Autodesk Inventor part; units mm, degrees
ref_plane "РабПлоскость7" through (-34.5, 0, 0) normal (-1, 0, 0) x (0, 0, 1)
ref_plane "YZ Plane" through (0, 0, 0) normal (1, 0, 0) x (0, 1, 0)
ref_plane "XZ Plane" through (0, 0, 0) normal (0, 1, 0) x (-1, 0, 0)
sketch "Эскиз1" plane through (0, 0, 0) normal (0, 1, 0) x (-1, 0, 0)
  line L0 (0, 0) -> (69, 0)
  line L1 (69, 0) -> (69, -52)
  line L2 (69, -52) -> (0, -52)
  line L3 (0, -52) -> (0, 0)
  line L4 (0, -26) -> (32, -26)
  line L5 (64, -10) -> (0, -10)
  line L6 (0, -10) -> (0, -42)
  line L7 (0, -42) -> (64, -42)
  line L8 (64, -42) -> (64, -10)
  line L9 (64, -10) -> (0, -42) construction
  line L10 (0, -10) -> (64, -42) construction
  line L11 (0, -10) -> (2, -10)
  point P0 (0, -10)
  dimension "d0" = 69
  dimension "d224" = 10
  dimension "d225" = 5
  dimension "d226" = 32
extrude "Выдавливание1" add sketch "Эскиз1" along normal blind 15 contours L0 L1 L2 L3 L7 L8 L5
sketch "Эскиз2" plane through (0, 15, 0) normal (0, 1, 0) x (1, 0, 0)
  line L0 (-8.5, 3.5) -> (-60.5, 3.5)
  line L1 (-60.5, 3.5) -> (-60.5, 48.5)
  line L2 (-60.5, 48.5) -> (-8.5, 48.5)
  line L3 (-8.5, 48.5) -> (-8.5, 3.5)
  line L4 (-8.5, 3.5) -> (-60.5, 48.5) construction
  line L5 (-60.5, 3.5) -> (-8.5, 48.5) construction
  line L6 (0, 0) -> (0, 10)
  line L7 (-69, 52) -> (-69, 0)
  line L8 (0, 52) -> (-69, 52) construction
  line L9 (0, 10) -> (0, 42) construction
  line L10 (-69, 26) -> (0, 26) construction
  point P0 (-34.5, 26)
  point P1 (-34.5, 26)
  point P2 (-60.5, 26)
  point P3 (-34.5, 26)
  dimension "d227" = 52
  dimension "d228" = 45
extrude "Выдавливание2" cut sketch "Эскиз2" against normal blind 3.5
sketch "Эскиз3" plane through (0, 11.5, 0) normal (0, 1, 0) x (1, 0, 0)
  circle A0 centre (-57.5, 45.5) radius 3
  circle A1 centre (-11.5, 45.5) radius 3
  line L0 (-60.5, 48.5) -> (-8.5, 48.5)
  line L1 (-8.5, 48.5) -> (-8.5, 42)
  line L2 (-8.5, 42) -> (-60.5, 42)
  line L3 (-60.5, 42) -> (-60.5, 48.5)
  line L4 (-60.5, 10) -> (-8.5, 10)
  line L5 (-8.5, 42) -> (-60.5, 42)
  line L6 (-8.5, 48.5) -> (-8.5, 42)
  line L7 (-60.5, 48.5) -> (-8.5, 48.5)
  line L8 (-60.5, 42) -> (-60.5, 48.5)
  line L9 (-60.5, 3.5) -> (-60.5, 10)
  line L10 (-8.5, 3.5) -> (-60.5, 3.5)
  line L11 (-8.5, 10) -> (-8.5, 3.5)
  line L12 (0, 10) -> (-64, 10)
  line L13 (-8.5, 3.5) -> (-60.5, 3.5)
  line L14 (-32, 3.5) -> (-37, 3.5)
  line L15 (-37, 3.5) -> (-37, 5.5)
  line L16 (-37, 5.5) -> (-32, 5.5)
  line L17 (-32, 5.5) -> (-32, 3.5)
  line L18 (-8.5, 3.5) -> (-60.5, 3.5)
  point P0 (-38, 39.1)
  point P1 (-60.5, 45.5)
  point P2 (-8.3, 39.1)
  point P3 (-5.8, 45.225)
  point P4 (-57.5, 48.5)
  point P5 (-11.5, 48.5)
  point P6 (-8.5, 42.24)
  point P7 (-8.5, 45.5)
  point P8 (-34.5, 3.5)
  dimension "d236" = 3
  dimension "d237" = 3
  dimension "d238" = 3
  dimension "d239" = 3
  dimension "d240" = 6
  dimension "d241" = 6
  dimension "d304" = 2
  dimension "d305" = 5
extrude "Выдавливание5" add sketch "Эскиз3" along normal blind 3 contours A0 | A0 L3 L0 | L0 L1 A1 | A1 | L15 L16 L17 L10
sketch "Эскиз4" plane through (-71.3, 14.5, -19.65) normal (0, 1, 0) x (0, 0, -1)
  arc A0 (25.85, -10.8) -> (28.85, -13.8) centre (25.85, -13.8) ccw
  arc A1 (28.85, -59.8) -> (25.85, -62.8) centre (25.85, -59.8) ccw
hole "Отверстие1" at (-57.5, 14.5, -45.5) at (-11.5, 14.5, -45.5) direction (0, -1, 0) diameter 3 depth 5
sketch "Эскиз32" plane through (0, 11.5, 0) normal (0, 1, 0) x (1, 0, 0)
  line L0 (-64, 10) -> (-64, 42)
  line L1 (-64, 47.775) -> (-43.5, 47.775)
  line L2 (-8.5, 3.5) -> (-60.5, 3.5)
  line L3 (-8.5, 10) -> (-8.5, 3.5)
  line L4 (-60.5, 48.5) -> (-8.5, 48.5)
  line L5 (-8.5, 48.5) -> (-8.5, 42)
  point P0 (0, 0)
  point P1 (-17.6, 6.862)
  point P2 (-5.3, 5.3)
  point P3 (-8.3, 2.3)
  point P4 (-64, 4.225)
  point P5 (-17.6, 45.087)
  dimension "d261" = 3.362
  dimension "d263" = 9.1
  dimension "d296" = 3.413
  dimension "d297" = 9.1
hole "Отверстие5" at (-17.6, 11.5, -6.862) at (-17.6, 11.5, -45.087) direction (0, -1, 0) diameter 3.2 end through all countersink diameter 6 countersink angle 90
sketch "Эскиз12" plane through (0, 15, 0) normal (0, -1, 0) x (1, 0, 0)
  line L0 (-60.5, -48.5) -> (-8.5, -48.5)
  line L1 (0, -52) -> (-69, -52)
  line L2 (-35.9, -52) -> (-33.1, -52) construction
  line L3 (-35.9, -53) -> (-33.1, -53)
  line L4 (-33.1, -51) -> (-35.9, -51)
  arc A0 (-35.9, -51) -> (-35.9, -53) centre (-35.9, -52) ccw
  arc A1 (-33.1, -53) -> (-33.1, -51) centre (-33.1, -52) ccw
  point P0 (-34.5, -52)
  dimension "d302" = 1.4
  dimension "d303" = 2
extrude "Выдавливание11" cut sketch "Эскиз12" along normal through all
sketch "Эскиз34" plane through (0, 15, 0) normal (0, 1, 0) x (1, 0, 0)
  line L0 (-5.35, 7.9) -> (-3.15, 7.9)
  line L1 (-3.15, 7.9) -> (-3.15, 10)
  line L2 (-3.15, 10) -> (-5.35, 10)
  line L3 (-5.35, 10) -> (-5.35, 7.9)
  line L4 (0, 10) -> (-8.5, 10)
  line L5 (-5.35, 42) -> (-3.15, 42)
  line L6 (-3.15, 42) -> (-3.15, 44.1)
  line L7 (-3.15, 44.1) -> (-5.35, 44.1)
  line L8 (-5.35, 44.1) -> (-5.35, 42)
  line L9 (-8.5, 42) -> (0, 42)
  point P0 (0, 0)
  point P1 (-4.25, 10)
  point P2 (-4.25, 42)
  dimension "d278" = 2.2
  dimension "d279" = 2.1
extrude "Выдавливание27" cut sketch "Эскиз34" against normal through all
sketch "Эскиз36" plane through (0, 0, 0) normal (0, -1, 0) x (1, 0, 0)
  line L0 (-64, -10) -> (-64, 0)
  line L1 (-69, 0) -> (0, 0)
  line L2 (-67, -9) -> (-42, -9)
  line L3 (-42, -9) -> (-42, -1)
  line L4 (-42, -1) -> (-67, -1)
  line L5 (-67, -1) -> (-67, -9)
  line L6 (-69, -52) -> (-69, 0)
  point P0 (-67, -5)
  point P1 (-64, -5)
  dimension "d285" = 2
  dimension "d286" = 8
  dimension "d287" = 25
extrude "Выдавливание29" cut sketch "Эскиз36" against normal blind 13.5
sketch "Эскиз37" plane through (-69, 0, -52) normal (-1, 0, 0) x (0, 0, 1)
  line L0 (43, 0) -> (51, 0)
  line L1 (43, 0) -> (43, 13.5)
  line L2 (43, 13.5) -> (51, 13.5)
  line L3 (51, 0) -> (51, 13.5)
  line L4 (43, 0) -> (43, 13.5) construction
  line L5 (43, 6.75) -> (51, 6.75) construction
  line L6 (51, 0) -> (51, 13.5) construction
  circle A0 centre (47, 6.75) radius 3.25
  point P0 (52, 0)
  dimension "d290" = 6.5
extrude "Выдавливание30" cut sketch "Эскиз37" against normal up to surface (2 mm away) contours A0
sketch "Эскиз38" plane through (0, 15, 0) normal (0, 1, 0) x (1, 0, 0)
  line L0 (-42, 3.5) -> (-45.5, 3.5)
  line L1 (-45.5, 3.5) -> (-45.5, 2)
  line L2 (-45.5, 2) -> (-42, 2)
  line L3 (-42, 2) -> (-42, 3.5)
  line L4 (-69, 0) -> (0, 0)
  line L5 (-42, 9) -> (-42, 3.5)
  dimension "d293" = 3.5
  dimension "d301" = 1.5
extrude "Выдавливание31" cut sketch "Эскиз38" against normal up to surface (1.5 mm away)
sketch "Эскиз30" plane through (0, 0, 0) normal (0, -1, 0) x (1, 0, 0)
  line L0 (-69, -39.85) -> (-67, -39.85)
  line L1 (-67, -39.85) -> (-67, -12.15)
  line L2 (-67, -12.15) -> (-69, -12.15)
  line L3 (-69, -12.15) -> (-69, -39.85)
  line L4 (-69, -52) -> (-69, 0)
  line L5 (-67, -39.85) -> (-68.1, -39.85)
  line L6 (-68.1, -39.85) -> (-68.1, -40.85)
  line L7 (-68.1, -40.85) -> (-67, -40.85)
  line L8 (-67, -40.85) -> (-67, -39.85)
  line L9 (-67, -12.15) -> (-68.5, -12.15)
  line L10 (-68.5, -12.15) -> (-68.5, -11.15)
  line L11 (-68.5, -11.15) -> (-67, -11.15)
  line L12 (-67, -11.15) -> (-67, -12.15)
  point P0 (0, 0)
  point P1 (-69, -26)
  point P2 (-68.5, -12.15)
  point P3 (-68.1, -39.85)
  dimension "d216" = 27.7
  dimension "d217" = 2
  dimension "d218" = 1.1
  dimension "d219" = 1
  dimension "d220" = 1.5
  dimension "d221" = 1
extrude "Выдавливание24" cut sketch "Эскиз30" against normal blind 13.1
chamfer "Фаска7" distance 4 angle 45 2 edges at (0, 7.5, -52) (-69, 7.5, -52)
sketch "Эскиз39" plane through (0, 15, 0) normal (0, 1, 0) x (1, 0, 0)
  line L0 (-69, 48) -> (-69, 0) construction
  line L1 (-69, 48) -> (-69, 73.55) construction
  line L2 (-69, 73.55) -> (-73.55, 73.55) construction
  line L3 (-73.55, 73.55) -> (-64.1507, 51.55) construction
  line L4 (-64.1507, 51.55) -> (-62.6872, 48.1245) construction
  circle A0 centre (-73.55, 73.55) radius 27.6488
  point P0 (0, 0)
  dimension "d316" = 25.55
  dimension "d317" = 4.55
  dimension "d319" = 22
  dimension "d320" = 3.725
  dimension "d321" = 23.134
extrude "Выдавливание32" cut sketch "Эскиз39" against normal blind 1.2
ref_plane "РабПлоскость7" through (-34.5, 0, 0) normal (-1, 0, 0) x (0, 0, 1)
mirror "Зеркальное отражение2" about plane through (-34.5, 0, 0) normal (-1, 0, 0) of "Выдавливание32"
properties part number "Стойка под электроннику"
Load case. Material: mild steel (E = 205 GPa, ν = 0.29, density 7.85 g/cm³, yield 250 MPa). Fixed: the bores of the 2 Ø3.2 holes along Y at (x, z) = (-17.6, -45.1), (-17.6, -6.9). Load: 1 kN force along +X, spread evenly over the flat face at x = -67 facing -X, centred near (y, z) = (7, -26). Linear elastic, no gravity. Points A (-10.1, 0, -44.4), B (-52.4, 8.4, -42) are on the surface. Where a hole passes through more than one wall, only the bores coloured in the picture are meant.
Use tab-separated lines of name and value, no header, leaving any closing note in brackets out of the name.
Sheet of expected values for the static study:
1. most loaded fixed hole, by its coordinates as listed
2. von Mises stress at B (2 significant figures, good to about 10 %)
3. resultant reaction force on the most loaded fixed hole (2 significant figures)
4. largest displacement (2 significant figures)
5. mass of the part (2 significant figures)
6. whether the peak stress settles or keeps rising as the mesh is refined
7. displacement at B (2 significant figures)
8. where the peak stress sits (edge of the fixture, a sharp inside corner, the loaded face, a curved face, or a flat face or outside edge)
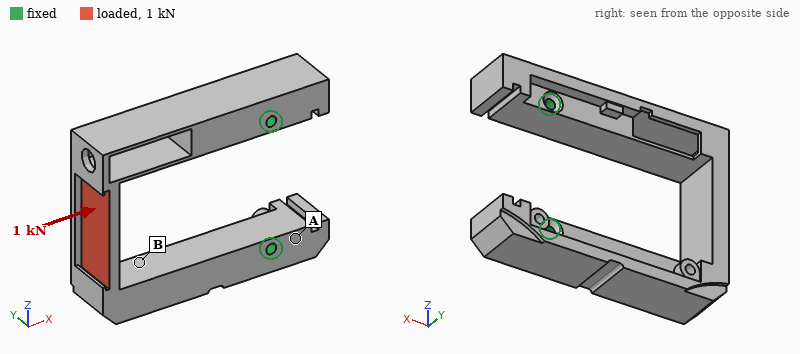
most loaded fixed hole, by its coordinates as listed	(-17.6, -45.1)
von Mises stress at B	29 MPa
resultant reaction force on the most loaded fixed hole	550 N
largest displacement	42 µm
mass of the part	130 g
whether the peak stress settles or keeps rising as the mesh is refined	keeps rising
displacement at B	12 µm
where the peak stress sits	a sharp inside corner
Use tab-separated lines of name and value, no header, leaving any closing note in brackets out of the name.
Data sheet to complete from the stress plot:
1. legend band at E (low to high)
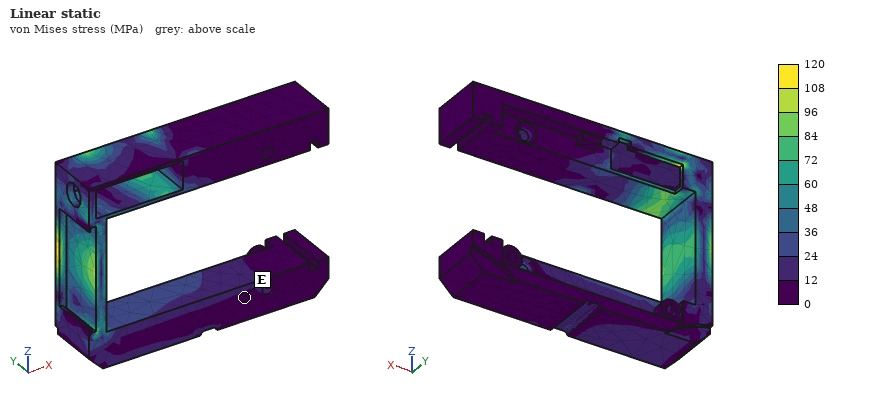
legend band at E	0 to 12 MPa
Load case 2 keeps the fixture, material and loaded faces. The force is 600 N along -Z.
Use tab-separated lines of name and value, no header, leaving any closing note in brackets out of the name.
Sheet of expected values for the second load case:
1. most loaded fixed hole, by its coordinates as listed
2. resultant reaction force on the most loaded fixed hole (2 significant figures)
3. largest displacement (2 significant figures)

most loaded fixed hole, by its coordinates as listed	(-17.6, -45.1)
resultant reaction force on the most loaded fixed hole	510 N
largest displacement	0.11 mm
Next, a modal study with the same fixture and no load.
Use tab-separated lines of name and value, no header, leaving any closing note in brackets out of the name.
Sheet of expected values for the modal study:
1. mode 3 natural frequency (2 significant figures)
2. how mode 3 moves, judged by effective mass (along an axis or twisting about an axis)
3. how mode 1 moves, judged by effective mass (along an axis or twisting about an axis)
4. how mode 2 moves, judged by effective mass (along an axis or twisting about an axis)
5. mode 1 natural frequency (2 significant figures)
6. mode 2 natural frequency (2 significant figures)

mode 3 natural frequency	4800 Hz
how mode 3 moves, judged by effective mass	twisting about X
how mode 1 moves, judged by effective mass	along Z
how mode 2 moves, judged by effective mass	along Y
mode 1 natural frequency	2100 Hz
mode 2 natural frequency	3100 Hz
